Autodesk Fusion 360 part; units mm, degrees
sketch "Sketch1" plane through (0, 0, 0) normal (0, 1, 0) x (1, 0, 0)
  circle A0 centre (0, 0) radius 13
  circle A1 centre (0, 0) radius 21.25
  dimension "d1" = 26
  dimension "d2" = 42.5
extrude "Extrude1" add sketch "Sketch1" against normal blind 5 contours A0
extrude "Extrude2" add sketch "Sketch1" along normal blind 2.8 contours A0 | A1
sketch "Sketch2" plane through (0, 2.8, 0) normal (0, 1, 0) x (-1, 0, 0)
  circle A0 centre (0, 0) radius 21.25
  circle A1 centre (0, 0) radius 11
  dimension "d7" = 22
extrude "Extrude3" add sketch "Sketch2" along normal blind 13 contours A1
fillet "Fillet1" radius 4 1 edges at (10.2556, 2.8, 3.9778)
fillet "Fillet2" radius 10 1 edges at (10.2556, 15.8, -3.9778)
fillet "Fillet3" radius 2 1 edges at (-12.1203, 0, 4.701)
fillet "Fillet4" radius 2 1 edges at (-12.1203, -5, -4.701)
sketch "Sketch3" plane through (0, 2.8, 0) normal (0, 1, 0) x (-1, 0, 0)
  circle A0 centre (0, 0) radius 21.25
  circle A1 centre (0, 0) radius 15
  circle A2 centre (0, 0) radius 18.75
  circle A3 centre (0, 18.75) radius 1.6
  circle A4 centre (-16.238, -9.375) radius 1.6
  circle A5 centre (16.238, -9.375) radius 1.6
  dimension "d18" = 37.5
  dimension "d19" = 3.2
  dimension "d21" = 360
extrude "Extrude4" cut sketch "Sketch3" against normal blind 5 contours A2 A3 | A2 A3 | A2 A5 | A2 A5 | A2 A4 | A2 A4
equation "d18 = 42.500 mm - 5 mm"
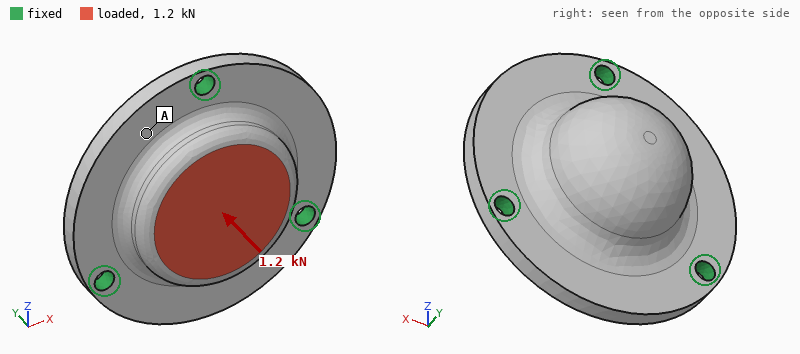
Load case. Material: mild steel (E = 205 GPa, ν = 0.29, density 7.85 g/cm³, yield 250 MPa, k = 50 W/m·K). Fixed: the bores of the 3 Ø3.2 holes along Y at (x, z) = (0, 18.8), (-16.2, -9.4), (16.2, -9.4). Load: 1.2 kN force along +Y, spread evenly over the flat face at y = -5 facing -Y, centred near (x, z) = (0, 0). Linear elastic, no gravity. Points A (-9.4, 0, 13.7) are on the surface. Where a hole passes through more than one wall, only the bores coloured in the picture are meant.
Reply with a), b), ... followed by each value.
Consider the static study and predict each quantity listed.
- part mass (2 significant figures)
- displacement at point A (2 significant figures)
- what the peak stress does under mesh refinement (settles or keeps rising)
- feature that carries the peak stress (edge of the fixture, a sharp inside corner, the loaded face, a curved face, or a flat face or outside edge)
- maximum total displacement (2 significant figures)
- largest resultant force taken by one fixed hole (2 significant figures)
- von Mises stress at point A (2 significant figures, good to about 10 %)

a) 83 g
b) 2.4 µm
c) keeps rising
d) edge of the fixture
e) 2.9 µm
f) 400 N
g) 10 MPa
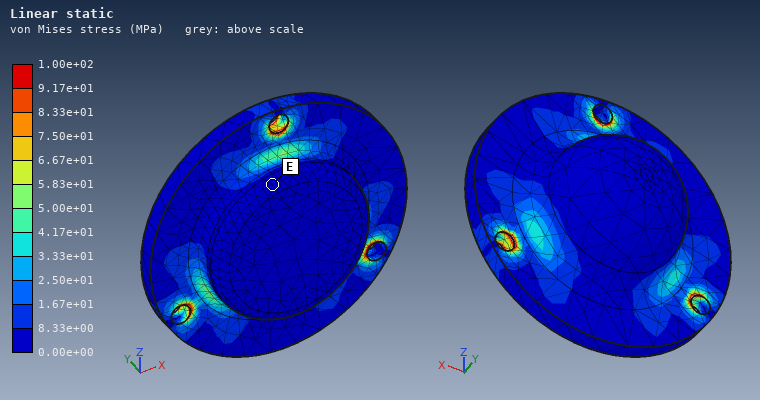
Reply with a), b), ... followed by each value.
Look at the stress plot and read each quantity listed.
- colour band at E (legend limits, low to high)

a) 0.00e+00 to 8.33e+00 MPa
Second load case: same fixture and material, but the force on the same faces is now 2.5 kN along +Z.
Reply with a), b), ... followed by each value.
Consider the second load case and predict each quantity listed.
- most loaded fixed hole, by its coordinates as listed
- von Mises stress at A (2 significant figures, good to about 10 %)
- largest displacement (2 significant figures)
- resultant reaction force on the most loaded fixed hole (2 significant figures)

a) (0, 18.8)
b) 20 MPa
c) 6.5 µm
d) 1.2 kN
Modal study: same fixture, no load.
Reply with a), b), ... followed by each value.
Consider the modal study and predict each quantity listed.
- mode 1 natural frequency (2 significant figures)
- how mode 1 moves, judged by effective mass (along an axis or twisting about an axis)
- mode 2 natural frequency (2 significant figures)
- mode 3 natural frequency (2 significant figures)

a) 12 kHz
b) along Y
c) 15 kHz
d) 15 kHz
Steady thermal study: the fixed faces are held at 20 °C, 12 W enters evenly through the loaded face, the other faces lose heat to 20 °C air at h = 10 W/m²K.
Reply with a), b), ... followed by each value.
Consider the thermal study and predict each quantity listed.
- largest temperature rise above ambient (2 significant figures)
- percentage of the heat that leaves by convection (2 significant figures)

a) 18 K
b) 3.2 %
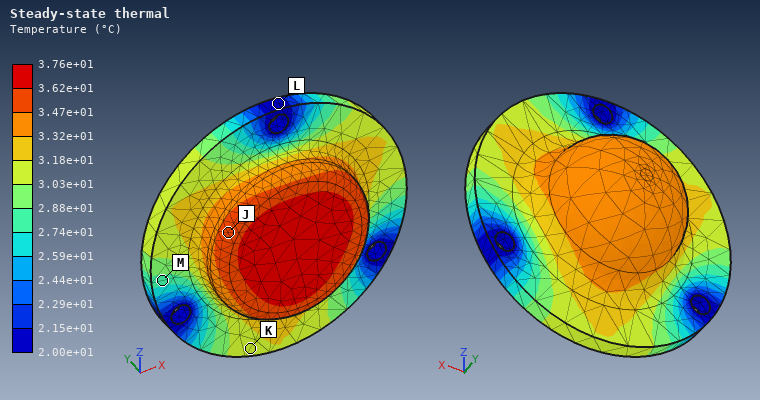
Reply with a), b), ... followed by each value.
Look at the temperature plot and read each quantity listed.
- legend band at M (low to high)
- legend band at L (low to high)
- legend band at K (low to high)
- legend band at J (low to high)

a) 2.74e+01 to 2.88e+01 °C
b) 2.00e+01 to 2.15e+01 °C
c) 3.03e+01 to 3.18e+01 °C
d) 3.47e+01 to 3.62e+01 °C
